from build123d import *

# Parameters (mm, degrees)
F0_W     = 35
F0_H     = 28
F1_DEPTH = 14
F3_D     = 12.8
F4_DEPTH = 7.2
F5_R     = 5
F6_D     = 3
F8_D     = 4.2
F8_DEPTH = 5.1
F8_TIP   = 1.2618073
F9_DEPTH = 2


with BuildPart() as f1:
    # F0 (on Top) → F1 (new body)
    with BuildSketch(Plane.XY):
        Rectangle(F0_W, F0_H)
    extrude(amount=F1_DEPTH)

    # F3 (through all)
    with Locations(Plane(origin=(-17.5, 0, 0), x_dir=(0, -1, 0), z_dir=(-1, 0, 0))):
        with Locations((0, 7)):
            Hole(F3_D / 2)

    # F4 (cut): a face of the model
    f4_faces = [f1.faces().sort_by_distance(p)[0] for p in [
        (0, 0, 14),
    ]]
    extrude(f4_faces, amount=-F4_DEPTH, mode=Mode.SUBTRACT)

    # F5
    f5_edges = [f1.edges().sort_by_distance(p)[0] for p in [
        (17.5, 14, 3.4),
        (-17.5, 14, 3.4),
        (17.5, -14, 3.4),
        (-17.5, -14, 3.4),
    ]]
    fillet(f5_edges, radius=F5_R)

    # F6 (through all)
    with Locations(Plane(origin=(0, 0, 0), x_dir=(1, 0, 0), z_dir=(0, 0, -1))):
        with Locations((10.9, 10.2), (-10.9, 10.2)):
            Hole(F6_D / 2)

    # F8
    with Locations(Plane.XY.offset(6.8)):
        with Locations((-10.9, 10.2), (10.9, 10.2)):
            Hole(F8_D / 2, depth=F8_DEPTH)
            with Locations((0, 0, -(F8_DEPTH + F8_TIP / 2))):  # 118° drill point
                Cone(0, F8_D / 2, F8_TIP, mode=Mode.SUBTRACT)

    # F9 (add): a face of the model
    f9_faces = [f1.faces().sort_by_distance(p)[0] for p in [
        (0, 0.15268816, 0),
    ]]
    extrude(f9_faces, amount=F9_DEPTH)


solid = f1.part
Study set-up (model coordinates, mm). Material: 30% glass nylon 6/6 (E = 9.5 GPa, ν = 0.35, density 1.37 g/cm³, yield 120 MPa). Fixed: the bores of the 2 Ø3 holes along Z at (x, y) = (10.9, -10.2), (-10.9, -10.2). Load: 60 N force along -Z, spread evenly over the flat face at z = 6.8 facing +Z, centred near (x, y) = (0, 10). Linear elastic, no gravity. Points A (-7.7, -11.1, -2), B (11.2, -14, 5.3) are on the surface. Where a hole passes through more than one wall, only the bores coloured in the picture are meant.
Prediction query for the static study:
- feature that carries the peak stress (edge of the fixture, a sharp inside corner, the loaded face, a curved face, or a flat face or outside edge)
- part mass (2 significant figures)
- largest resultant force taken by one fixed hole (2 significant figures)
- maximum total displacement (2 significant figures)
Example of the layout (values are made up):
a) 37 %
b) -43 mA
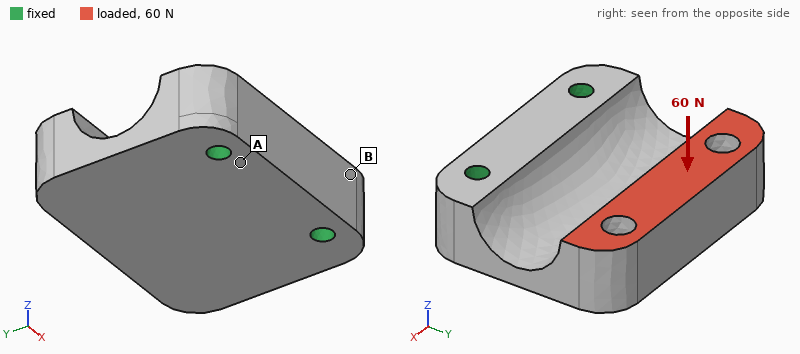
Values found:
a) a curved face
b) 8.2 g
c) 30 N
d) 0.15 mm
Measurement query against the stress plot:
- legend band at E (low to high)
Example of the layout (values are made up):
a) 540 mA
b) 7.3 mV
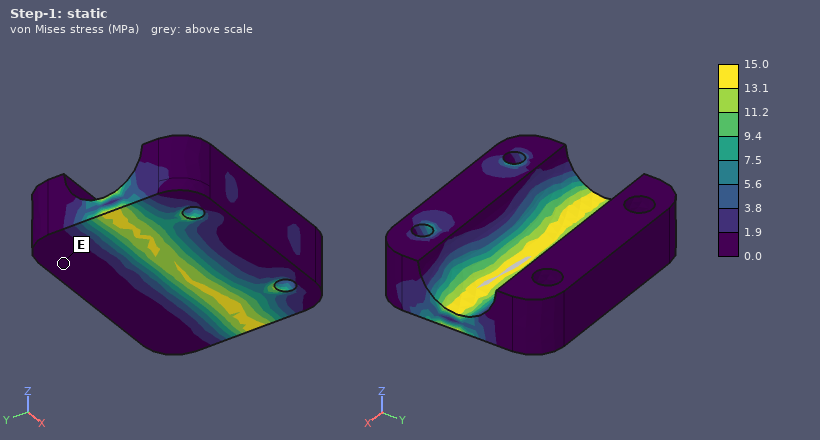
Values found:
a) 0.0 to 1.9 MPa
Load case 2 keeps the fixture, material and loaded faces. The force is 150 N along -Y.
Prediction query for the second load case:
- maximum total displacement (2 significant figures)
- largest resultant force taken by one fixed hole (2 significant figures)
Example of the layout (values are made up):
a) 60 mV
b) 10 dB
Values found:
a) 0.24 mm
b) 77 N
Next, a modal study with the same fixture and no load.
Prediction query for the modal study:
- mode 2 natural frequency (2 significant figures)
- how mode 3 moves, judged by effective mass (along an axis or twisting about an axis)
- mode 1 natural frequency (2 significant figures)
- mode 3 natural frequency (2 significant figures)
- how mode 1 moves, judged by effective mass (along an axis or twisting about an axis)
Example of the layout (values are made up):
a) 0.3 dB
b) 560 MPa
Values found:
a) 5400 Hz
b) along X
c) 2100 Hz
d) 9000 Hz
e) along Z
